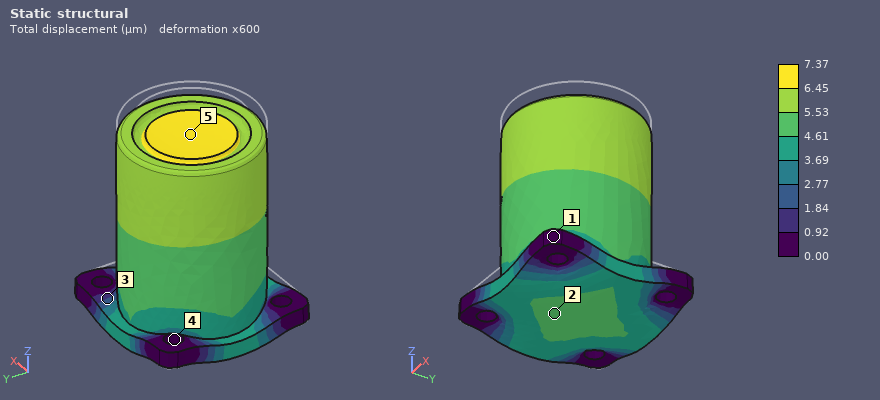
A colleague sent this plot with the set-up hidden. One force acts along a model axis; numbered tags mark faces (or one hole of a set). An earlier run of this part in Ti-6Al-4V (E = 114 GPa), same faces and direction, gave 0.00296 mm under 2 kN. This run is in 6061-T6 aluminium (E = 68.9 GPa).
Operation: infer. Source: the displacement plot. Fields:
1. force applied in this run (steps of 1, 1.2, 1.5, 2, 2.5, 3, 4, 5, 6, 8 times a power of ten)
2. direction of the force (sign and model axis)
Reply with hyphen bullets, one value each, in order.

- 3 kN
- -Z
